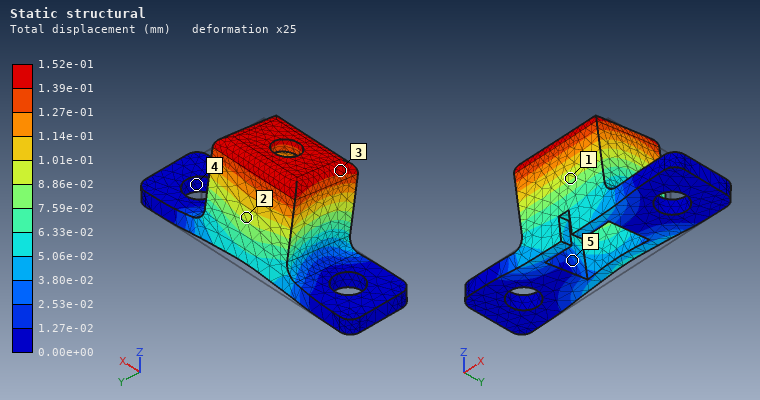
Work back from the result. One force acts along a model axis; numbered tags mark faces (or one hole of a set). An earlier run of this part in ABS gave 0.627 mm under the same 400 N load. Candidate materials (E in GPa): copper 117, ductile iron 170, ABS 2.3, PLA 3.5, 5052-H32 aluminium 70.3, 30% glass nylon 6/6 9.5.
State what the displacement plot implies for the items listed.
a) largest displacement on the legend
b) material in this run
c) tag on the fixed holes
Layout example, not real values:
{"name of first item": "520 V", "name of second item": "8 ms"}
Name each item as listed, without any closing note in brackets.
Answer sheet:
{"largest displacement on the legend": "1.52e-01 mm", "material in this run": "30% glass nylon 6/6", "tag on the fixed holes": "4"}
